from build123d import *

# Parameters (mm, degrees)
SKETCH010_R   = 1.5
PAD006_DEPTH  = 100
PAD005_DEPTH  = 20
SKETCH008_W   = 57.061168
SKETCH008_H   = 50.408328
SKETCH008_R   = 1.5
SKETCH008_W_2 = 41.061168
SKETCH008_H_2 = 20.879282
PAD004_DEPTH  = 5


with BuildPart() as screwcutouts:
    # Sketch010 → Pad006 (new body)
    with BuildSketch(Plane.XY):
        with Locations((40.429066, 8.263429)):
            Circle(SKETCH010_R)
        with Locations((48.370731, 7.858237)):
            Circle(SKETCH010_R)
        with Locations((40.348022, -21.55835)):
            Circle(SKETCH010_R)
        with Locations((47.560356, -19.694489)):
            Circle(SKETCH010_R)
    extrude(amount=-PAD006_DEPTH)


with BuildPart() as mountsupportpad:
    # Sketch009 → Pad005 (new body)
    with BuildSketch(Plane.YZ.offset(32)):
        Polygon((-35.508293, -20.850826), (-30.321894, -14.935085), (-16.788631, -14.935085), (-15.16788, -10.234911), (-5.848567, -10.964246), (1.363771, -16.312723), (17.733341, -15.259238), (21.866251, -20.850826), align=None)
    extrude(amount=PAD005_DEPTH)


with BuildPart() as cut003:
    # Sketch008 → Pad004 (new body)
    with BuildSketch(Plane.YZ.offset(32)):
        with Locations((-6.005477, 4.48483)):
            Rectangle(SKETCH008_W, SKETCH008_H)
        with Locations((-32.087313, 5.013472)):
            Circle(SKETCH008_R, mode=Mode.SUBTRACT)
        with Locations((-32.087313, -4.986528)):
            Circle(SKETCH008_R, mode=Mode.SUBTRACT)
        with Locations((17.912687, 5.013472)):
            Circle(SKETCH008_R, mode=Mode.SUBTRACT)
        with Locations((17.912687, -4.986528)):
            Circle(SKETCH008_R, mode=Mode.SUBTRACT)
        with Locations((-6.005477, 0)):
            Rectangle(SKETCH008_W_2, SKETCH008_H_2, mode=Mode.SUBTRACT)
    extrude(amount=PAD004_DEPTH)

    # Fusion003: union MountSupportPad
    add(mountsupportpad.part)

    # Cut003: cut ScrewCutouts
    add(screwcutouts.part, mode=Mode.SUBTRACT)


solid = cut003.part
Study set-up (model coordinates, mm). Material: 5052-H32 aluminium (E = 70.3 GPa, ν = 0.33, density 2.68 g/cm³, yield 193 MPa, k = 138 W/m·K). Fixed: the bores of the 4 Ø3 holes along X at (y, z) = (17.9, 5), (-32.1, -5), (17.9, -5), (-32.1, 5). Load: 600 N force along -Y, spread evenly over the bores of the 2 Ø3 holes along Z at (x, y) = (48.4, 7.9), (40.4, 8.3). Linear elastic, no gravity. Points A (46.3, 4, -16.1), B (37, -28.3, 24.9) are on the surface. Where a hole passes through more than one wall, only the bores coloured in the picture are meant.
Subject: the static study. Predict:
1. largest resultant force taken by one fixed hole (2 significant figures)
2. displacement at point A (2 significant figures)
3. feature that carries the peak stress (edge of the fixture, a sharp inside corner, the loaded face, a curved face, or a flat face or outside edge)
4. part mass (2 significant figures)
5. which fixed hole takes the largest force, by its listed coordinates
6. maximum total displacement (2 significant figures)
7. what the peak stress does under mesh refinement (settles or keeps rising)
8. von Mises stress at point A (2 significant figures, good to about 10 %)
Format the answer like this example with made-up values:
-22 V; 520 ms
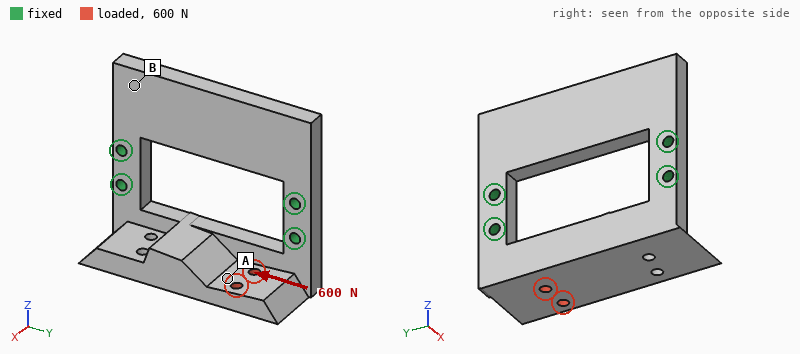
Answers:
410 N; 10 µm; edge of the fixture; 40 g; (-32.1, -5); 14 µm; keeps rising; 7.1 MPa
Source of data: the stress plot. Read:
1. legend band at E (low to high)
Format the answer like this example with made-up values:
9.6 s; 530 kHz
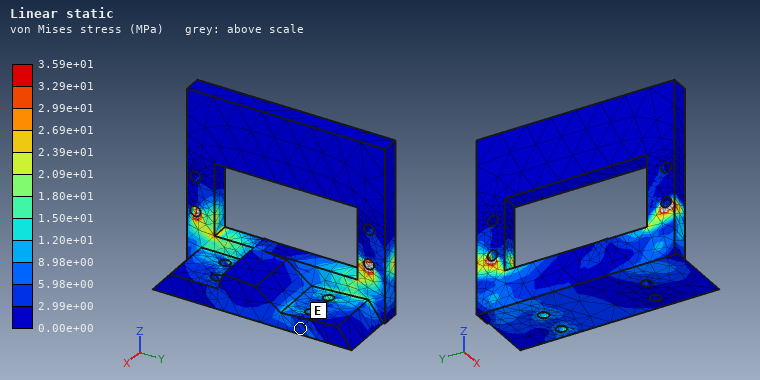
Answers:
2.99e+00 to 5.98e+00 MPa
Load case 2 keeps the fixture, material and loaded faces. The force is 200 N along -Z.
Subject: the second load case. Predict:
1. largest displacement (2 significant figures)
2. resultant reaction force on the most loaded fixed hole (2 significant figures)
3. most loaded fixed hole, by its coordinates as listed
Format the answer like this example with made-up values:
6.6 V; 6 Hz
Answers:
46 µm; 170 N; (17.9, -5)
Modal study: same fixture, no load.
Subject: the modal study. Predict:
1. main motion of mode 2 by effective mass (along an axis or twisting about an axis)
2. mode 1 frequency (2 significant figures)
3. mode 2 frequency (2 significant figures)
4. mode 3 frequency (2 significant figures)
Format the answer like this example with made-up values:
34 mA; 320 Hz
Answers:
along X; 3100 Hz; 3400 Hz; 7800 Hz
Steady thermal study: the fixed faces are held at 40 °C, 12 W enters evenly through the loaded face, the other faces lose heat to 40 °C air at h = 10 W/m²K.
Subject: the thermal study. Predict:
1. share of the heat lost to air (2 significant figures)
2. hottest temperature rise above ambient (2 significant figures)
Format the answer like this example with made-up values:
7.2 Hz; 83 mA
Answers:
4.0 %; 21 K
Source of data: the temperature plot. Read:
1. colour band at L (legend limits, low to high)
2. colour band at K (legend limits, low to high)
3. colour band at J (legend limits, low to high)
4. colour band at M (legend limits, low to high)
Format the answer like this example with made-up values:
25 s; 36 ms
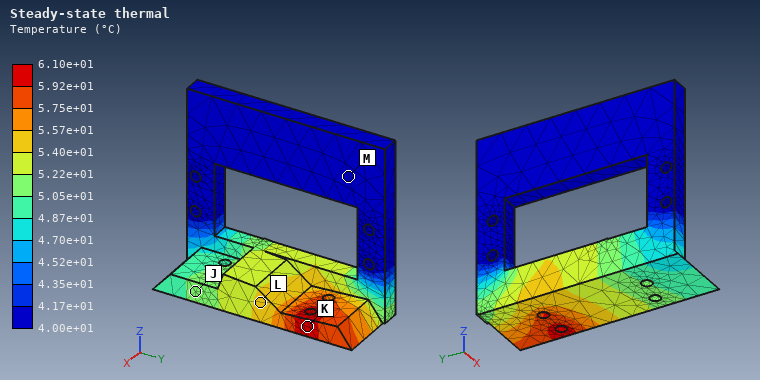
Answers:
5.40e+01 to 5.57e+01 °C; 5.92e+01 to 6.10e+01 °C; 5.05e+01 to 5.22e+01 °C; 4.00e+01 to 4.17e+01 °C
